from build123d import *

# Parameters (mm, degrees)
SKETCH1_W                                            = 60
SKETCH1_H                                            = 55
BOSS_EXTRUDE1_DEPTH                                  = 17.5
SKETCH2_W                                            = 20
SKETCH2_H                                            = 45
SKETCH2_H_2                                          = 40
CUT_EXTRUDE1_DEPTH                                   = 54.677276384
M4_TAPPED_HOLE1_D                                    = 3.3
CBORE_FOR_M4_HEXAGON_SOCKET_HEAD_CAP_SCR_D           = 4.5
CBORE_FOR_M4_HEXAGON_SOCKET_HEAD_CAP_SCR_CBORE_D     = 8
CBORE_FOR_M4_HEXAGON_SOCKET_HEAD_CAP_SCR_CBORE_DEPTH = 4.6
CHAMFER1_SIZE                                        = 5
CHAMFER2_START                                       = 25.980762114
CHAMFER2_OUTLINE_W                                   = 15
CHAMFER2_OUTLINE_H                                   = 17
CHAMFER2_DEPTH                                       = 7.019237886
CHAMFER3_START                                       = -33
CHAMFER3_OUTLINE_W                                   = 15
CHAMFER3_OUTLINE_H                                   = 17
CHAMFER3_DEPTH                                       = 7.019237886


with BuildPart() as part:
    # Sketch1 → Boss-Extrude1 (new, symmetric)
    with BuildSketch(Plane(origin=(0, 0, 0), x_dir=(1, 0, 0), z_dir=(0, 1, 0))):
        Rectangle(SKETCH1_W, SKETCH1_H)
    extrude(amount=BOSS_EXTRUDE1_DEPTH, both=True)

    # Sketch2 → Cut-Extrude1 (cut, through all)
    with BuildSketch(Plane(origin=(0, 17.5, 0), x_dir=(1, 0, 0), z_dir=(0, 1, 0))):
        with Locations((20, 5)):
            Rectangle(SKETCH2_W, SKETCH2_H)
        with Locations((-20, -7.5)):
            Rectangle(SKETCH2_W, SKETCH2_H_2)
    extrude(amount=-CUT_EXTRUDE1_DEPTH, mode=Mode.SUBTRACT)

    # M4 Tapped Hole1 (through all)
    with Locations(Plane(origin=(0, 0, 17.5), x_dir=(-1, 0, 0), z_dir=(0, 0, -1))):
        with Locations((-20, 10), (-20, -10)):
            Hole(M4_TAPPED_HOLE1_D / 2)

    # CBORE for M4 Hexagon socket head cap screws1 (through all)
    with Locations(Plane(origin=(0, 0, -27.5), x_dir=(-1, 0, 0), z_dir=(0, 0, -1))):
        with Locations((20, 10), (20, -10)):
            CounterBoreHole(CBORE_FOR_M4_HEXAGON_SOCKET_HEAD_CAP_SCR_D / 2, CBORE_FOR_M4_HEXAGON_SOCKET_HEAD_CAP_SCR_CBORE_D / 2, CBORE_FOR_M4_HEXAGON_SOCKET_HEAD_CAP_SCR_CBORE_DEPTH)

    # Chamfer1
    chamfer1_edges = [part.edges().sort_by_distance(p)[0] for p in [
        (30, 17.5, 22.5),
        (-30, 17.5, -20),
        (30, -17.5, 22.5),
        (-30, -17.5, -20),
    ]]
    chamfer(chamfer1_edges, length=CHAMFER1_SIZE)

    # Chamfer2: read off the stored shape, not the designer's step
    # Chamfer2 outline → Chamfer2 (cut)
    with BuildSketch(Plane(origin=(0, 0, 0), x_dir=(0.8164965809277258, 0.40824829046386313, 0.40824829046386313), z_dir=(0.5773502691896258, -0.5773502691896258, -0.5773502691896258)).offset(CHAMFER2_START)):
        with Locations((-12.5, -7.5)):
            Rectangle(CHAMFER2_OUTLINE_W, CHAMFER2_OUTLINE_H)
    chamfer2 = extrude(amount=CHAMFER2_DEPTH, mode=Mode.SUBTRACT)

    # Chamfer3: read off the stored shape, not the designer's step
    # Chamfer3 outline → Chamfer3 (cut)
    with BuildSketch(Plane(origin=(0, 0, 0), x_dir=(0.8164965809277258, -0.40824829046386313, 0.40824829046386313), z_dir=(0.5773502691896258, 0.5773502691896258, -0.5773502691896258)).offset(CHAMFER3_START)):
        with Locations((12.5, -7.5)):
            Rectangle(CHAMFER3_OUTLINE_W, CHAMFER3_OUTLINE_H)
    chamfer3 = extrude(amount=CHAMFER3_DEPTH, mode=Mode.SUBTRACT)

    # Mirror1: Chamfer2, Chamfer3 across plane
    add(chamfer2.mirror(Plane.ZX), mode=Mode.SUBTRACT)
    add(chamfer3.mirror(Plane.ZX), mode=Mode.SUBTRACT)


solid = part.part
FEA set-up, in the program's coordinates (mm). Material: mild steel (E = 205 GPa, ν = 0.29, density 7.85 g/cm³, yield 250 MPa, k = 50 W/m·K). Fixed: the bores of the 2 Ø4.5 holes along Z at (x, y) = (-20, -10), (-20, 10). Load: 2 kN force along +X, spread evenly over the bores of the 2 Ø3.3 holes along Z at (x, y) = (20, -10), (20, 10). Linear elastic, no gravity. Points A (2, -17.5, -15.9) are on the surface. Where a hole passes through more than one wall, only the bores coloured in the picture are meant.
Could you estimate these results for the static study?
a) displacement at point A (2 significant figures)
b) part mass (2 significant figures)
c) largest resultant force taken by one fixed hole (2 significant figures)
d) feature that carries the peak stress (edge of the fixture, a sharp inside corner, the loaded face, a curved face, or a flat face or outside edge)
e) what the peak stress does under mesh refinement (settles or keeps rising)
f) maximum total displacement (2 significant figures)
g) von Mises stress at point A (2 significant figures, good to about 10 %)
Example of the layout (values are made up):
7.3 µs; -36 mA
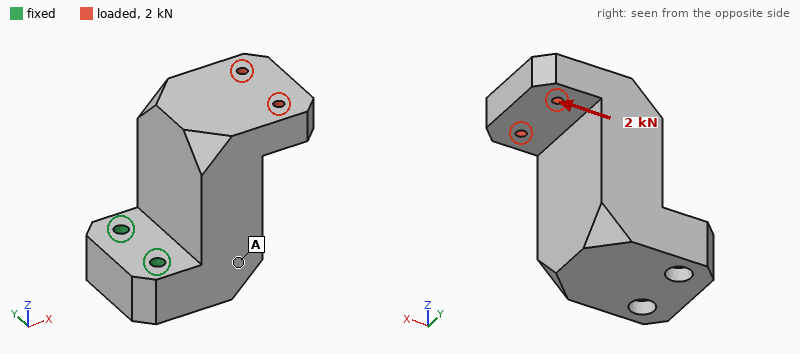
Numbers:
18 µm; 420 g; 1.1 kN; edge of the fixture; keeps rising; 82 µm; 23 MPa
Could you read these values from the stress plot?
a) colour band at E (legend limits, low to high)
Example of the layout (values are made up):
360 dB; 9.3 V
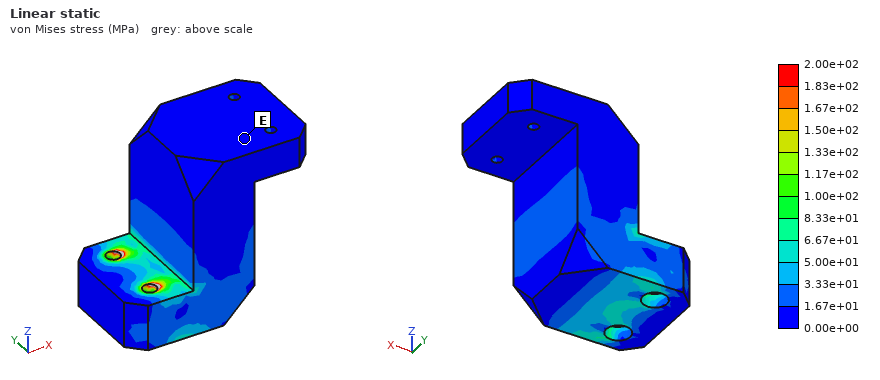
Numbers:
0.00e+00 to 1.67e+01 MPa
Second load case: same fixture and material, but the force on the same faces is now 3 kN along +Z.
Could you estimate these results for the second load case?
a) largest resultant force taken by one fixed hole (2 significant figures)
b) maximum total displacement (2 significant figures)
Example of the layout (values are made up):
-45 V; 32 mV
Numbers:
1.5 kN; 0.12 mm
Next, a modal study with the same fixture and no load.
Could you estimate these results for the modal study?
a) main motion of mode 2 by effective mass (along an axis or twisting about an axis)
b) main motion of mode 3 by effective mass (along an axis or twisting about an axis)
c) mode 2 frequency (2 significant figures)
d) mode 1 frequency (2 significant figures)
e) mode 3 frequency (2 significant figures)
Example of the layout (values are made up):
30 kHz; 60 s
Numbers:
along Y; twisting about Z; 3500 Hz; 2100 Hz; 8300 Hz
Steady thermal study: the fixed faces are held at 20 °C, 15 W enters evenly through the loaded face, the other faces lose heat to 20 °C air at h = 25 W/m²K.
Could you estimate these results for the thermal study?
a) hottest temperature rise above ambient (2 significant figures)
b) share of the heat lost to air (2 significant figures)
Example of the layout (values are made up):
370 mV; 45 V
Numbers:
35 K; 25 %
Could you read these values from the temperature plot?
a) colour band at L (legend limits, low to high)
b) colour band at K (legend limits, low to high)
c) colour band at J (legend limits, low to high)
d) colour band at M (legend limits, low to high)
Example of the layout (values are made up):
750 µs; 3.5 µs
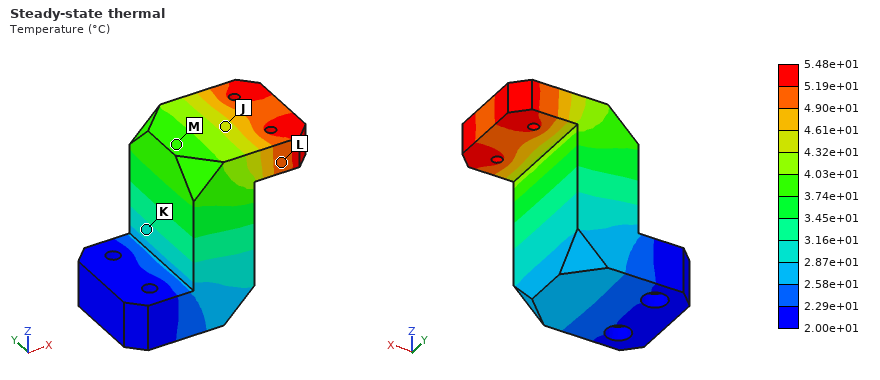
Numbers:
4.90e+01 to 5.19e+01 °C; 2.87e+01 to 3.16e+01 °C; 4.32e+01 to 4.61e+01 °C; 3.74e+01 to 4.03e+01 °C
